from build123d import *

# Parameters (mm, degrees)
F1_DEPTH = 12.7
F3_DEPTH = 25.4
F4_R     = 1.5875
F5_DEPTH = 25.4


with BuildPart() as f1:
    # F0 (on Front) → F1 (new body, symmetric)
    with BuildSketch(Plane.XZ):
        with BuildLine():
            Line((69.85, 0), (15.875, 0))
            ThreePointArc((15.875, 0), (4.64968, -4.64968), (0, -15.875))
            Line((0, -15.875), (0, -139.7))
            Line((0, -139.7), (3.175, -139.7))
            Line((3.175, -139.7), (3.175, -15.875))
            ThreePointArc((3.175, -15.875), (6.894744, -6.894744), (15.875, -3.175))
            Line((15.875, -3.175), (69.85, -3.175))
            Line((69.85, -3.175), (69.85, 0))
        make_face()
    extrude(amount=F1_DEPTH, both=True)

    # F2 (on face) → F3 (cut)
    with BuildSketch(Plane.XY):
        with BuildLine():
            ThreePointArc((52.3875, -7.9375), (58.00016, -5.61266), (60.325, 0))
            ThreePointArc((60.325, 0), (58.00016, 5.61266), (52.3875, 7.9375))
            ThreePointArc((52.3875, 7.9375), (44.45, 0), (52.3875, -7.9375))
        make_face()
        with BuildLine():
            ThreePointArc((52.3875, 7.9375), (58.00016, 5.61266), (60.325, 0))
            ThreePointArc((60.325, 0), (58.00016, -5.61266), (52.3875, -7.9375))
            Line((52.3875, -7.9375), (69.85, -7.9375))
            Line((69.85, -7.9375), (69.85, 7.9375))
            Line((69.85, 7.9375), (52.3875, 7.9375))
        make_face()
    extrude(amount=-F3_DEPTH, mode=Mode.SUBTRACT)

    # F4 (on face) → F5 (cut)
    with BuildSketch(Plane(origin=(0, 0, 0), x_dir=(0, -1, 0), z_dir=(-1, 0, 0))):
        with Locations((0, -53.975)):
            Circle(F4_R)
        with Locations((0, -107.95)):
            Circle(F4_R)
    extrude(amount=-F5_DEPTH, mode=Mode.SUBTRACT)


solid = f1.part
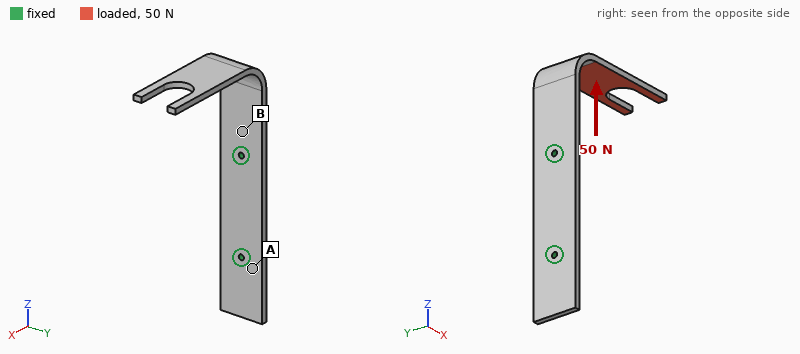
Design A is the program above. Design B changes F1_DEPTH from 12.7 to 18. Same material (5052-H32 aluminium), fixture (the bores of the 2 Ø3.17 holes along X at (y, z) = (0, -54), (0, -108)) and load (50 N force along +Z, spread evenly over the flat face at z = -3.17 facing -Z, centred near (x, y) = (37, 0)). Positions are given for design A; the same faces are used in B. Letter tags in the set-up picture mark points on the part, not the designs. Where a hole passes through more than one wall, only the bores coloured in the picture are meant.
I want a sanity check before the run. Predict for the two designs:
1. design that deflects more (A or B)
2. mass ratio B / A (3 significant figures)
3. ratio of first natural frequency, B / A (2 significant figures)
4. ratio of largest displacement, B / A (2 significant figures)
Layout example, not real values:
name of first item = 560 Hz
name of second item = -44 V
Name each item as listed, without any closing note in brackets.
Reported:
design that deflects more = A
mass ratio B / A = 1.45
ratio of first natural frequency, B / A = 0.91
ratio of largest displacement, B / A = 0.76
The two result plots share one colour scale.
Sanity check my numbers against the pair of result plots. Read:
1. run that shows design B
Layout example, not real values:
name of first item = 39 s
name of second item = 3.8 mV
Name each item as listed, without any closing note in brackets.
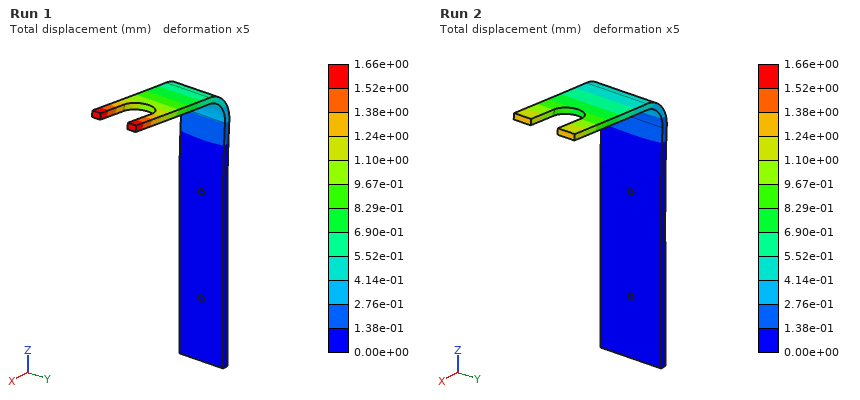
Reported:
run that shows design B = Run 2
